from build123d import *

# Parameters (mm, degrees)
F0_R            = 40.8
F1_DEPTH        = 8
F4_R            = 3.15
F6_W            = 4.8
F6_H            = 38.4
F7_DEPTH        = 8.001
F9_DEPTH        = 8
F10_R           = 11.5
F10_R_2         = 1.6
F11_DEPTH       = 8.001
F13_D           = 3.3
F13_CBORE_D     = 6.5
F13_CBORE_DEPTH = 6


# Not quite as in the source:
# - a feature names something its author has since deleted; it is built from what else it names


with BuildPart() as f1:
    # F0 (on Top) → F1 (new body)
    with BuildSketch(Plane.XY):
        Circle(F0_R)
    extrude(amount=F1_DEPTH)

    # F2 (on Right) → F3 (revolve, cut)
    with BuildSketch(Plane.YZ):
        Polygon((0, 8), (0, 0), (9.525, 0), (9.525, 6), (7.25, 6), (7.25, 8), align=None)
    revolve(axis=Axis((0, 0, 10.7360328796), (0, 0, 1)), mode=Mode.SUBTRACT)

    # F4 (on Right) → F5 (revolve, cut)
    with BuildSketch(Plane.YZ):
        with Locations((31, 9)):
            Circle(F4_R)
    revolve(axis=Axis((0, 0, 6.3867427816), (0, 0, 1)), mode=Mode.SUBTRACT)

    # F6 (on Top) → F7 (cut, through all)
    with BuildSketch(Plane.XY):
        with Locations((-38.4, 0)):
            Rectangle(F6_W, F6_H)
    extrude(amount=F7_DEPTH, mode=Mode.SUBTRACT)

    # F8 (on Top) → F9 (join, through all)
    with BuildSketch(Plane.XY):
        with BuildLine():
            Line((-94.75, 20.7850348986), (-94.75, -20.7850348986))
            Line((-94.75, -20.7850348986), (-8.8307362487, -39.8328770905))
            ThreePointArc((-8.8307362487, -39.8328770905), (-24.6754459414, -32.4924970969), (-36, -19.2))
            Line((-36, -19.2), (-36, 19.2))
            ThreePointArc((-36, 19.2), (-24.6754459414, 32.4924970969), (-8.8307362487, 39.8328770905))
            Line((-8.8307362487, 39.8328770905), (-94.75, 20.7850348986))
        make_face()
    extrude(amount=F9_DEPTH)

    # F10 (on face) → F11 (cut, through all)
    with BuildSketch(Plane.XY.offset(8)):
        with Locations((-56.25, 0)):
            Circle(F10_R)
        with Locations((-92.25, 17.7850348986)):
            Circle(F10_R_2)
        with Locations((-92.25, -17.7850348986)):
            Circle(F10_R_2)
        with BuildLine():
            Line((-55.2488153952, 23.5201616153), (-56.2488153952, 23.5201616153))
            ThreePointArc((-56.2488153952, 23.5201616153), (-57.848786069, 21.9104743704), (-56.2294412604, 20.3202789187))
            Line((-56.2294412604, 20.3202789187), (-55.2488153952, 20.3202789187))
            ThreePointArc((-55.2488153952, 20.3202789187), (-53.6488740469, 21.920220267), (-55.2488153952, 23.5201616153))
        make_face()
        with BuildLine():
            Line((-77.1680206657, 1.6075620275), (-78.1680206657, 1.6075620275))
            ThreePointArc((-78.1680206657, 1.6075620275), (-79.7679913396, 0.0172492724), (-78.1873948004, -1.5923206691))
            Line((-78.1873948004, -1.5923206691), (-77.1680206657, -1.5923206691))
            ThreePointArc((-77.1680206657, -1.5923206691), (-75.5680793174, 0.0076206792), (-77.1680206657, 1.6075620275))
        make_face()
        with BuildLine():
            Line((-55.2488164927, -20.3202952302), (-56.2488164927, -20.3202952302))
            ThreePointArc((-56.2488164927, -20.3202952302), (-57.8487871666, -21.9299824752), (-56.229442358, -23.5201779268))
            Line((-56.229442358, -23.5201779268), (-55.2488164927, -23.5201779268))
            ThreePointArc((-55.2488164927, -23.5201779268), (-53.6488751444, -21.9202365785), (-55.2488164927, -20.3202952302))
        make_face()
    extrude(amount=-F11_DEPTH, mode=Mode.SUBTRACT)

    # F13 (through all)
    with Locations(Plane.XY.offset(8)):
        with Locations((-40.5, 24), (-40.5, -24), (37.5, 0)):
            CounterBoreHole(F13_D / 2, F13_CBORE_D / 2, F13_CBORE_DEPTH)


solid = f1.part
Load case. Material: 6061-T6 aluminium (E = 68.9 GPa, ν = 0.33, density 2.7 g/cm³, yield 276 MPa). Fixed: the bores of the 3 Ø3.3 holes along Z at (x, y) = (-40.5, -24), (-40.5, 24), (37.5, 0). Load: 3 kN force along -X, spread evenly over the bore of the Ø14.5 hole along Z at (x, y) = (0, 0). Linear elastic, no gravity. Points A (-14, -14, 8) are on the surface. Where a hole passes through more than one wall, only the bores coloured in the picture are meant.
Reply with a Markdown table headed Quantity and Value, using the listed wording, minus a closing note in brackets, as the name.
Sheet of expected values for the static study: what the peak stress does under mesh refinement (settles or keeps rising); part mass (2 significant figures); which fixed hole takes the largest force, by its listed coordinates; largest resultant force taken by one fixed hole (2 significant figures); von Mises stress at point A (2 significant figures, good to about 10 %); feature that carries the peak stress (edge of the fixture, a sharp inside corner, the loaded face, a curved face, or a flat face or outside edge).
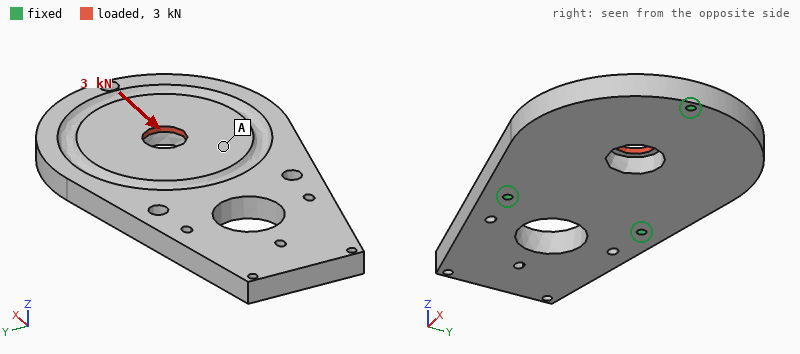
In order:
| Quantity | Value |
|---|---|
| what the peak stress does under mesh refinement | keeps rising |
| part mass | 160 g |
| which fixed hole takes the largest force, by its listed coordinates | (37.5, 0) |
| largest resultant force taken by one fixed hole | 1.1 kN |
| von Mises stress at point A | 6.7 MPa |
| feature that carries the peak stress | edge of the fixture |
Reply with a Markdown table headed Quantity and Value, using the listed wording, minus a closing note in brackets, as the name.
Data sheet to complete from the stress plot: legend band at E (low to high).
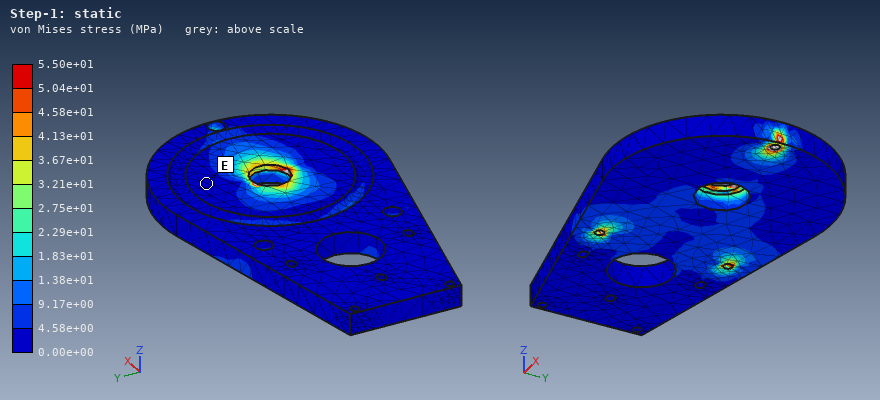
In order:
| Quantity | Value |
|---|---|
| legend band at E | 0.00e+00 to 4.58e+00 MPa |
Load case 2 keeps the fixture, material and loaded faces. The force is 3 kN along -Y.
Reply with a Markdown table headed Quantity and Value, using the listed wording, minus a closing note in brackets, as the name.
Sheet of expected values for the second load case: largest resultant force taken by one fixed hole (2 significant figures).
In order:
| Quantity | Value |
|---|---|
| largest resultant force taken by one fixed hole | 1.2 kN |
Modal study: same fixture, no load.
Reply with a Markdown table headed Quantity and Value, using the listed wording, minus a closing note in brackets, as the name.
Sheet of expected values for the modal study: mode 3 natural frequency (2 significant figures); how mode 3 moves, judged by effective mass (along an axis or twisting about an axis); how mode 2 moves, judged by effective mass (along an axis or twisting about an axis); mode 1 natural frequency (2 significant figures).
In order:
| Quantity | Value |
|---|---|
| mode 3 natural frequency | 3300 Hz |
| how mode 3 moves, judged by effective mass | along Z |
| how mode 2 moves, judged by effective mass | twisting about X |
| mode 1 natural frequency | 1500 Hz |
